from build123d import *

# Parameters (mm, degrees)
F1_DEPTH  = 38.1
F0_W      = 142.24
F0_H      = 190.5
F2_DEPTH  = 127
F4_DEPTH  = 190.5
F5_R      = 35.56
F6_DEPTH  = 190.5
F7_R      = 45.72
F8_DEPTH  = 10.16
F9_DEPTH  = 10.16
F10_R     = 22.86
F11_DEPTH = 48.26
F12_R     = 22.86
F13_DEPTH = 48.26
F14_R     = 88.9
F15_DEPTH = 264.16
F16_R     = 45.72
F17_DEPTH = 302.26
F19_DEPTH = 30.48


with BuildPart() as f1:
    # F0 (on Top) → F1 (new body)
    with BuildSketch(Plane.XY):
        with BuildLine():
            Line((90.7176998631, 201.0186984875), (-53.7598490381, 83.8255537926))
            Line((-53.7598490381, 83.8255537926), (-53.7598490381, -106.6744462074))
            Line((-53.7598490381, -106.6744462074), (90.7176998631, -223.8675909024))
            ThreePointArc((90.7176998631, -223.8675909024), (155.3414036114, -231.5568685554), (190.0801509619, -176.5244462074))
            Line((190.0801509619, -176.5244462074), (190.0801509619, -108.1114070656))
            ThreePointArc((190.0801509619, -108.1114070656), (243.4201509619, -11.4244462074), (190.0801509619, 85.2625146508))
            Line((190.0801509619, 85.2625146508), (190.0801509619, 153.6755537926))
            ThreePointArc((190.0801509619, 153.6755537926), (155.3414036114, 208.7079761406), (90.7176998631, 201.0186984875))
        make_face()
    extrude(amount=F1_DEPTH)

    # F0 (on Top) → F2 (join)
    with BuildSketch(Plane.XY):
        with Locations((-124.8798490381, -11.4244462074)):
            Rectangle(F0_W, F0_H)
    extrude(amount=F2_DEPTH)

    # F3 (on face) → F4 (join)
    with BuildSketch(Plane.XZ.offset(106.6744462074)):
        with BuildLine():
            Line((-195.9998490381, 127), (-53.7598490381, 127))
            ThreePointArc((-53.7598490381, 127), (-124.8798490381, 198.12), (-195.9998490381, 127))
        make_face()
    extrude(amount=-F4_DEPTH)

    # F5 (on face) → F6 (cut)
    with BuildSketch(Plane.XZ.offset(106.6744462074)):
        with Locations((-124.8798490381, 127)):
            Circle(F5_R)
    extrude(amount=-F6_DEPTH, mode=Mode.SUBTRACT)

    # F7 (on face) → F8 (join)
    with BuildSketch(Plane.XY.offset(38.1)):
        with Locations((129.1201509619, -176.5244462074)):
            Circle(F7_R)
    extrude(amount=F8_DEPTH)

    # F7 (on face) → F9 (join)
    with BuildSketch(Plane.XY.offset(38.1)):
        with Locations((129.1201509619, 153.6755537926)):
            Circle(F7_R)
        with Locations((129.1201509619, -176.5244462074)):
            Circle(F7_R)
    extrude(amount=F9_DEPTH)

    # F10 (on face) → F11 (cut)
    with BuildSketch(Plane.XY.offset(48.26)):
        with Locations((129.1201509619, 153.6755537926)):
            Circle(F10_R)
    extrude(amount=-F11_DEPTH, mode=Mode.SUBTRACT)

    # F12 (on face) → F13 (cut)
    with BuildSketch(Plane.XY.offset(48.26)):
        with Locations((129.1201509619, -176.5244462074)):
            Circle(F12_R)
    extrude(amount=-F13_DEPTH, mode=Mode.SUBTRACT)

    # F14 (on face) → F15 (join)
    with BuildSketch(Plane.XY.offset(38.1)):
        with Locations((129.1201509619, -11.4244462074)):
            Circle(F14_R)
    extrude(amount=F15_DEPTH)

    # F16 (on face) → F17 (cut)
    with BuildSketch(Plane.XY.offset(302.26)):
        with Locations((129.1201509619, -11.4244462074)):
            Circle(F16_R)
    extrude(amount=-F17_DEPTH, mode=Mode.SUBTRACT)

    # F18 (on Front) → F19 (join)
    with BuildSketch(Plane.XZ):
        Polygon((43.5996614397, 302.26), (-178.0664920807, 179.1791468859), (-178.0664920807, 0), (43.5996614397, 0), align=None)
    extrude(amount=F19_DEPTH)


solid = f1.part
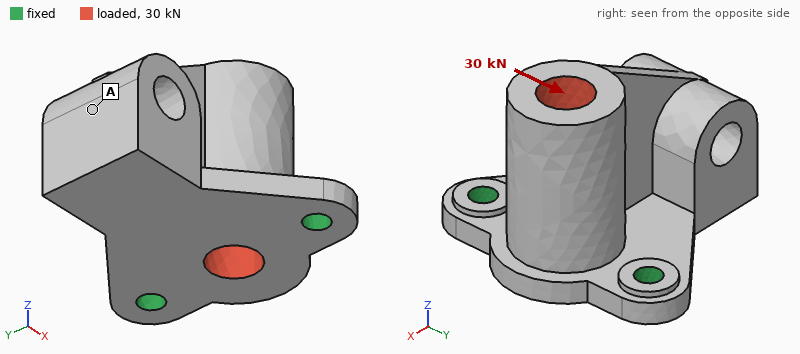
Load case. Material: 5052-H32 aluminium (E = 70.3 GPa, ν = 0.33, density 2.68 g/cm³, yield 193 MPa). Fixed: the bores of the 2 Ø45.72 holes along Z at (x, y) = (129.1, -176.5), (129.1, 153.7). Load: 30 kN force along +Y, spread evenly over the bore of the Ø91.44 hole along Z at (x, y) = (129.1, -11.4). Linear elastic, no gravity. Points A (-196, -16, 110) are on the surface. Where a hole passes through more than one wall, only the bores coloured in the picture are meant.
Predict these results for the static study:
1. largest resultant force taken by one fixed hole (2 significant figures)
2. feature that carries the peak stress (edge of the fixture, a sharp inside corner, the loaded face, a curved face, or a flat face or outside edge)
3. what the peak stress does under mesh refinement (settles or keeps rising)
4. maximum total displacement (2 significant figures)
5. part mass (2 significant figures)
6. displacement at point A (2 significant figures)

22 kN
edge of the fixture
keeps rising
0.10 mm
36 kg
0.022 mm
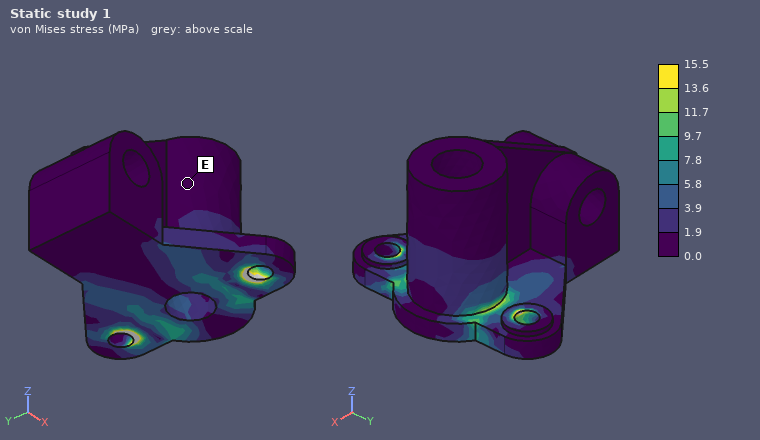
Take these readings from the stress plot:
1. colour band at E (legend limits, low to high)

0.0 to 1.9 MPa
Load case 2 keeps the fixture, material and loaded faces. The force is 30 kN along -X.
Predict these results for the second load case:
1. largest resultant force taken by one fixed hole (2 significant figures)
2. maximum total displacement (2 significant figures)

16 kN
0.53 mm
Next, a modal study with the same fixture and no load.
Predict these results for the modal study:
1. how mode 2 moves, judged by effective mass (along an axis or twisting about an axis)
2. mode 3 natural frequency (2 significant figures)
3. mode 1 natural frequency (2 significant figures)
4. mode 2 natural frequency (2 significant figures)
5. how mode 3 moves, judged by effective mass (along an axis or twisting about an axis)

along Y
990 Hz
220 Hz
650 Hz
along Z
